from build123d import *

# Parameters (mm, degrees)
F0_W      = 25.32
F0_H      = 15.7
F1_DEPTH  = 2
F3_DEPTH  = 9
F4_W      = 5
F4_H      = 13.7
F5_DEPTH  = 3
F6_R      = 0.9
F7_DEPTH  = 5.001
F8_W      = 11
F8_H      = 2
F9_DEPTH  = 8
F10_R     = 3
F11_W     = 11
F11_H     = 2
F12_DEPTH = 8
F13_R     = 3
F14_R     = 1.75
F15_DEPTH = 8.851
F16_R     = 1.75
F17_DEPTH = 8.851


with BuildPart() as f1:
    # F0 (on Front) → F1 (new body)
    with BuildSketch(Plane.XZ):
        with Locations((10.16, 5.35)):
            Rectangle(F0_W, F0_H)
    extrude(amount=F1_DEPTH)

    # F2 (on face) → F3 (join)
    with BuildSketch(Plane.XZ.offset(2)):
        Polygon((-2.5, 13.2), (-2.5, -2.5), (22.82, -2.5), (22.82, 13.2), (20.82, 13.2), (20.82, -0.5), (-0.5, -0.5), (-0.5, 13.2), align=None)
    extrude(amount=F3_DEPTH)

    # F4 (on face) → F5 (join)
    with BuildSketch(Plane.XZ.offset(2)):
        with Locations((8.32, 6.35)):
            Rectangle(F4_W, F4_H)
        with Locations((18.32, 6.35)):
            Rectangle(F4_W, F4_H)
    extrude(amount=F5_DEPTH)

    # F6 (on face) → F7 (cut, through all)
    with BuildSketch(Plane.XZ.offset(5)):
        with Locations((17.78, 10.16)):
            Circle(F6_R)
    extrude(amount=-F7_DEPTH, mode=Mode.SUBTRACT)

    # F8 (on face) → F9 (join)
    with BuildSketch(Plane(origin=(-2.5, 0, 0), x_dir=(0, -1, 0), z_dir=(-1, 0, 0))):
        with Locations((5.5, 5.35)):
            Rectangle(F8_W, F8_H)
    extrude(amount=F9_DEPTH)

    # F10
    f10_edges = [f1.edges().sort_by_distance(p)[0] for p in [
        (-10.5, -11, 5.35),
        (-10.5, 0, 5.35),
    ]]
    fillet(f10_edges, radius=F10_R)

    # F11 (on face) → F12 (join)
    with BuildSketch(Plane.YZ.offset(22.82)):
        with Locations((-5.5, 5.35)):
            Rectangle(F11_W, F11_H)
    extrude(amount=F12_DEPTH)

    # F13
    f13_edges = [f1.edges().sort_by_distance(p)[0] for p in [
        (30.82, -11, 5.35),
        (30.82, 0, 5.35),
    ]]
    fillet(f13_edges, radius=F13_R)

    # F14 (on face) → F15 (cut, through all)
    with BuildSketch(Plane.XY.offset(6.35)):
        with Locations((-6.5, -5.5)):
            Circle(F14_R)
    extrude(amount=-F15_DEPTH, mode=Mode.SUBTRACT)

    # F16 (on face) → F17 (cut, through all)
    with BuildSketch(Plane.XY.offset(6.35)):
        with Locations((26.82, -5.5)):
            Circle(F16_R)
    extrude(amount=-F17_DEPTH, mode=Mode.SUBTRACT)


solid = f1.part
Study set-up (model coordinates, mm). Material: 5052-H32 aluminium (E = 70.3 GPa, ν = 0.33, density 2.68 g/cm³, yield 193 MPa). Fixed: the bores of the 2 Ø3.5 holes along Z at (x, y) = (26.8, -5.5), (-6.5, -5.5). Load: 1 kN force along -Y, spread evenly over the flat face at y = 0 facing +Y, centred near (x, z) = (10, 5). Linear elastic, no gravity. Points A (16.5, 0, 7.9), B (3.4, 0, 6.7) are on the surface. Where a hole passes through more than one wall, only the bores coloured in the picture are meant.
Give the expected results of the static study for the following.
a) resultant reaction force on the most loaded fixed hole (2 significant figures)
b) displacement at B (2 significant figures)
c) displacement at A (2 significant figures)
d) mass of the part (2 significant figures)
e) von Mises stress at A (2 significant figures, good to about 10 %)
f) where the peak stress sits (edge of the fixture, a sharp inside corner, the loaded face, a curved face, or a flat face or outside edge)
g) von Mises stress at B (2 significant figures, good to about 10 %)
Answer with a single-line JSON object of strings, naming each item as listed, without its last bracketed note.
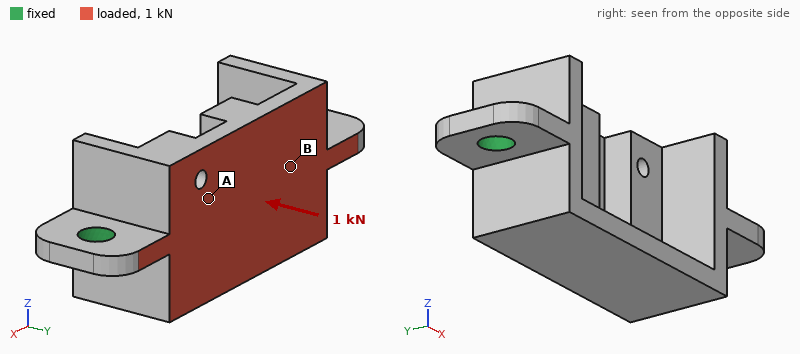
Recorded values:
{"resultant reaction force on the most loaded fixed hole": "630 N", "displacement at B": "19 µm", "displacement at A": "19 µm", "mass of the part": "6.5 g", "von Mises stress at A": "18 MPa", "where the peak stress sits": "edge of the fixture", "von Mises stress at B": "45 MPa"}
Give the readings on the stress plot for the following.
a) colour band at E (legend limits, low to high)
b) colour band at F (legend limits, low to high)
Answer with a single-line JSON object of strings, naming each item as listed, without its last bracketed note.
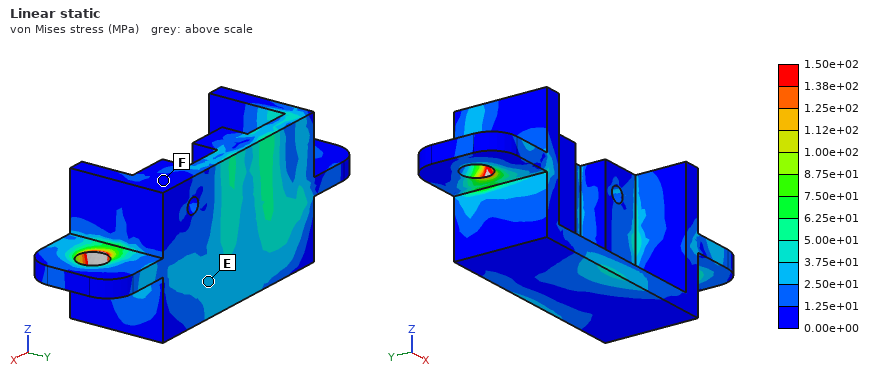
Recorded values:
{"colour band at E": "2.50e+01 to 3.75e+01 MPa", "colour band at F": "0.00e+00 to 1.25e+01 MPa"}
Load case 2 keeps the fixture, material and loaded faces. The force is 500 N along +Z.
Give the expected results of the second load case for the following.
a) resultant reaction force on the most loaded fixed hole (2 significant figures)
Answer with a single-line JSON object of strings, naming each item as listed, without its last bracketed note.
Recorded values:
{"resultant reaction force on the most loaded fixed hole": "250 N"}
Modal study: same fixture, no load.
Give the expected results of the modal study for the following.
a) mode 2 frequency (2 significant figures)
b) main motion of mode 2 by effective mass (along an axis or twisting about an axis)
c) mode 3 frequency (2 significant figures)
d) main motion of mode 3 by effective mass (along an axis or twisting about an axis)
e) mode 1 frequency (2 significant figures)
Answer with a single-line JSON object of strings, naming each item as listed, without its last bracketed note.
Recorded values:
{"mode 2 frequency": "16 kHz", "main motion of mode 2 by effective mass": "along Y", "mode 3 frequency": "17 kHz", "main motion of mode 3 by effective mass": "along Z", "mode 1 frequency": "8900 Hz"}
